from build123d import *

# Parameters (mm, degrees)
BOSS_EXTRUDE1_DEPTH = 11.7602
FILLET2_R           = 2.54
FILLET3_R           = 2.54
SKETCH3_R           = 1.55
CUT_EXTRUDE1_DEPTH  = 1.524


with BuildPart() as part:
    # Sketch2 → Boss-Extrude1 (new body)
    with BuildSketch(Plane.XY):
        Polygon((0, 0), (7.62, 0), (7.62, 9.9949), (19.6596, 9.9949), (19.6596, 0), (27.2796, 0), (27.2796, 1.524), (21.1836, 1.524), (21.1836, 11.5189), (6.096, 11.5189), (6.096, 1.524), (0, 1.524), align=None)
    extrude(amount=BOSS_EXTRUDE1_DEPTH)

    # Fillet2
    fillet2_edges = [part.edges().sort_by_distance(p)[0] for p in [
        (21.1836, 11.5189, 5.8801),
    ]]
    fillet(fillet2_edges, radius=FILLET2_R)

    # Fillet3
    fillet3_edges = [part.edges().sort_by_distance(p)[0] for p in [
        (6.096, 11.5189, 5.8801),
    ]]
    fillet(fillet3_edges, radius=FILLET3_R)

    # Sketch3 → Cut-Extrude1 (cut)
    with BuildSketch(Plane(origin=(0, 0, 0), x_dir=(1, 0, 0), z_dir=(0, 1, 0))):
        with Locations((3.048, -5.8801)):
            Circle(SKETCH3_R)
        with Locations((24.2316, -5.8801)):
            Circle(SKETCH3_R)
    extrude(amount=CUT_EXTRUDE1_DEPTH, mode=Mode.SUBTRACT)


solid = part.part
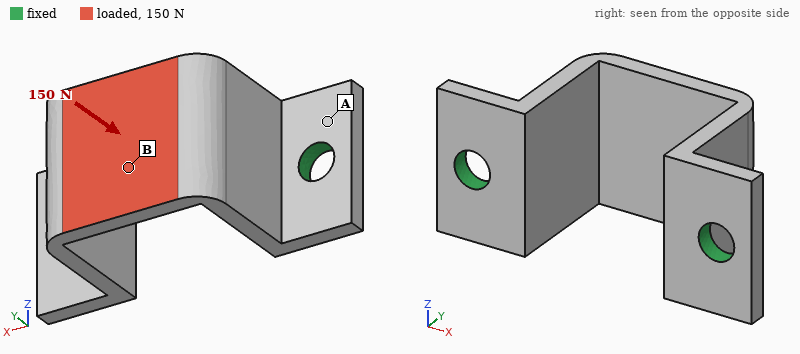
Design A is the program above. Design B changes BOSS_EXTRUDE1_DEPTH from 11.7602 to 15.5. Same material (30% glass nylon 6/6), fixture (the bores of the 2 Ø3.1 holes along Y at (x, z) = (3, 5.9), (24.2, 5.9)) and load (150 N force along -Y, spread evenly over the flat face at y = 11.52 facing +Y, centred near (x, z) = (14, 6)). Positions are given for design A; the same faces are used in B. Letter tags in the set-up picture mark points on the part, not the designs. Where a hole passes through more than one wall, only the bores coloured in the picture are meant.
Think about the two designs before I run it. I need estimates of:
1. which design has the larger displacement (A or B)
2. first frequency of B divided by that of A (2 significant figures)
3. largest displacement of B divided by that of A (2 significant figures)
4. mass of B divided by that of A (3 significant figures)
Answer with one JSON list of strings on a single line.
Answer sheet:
["B", "0.84", "1.4", "1.33"]
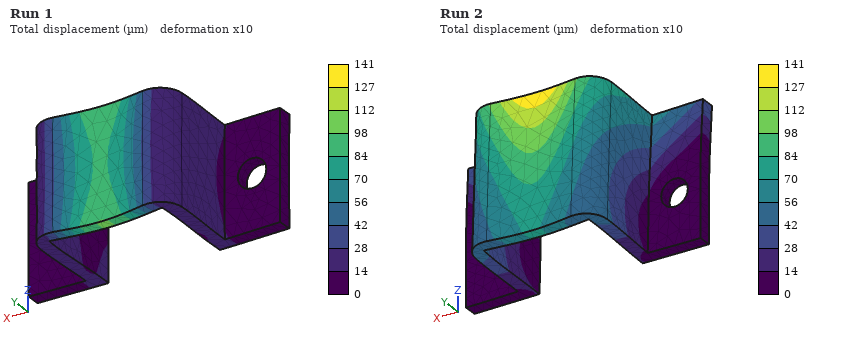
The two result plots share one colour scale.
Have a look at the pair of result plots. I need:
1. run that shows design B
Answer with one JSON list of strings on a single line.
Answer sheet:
["Run 2"]
